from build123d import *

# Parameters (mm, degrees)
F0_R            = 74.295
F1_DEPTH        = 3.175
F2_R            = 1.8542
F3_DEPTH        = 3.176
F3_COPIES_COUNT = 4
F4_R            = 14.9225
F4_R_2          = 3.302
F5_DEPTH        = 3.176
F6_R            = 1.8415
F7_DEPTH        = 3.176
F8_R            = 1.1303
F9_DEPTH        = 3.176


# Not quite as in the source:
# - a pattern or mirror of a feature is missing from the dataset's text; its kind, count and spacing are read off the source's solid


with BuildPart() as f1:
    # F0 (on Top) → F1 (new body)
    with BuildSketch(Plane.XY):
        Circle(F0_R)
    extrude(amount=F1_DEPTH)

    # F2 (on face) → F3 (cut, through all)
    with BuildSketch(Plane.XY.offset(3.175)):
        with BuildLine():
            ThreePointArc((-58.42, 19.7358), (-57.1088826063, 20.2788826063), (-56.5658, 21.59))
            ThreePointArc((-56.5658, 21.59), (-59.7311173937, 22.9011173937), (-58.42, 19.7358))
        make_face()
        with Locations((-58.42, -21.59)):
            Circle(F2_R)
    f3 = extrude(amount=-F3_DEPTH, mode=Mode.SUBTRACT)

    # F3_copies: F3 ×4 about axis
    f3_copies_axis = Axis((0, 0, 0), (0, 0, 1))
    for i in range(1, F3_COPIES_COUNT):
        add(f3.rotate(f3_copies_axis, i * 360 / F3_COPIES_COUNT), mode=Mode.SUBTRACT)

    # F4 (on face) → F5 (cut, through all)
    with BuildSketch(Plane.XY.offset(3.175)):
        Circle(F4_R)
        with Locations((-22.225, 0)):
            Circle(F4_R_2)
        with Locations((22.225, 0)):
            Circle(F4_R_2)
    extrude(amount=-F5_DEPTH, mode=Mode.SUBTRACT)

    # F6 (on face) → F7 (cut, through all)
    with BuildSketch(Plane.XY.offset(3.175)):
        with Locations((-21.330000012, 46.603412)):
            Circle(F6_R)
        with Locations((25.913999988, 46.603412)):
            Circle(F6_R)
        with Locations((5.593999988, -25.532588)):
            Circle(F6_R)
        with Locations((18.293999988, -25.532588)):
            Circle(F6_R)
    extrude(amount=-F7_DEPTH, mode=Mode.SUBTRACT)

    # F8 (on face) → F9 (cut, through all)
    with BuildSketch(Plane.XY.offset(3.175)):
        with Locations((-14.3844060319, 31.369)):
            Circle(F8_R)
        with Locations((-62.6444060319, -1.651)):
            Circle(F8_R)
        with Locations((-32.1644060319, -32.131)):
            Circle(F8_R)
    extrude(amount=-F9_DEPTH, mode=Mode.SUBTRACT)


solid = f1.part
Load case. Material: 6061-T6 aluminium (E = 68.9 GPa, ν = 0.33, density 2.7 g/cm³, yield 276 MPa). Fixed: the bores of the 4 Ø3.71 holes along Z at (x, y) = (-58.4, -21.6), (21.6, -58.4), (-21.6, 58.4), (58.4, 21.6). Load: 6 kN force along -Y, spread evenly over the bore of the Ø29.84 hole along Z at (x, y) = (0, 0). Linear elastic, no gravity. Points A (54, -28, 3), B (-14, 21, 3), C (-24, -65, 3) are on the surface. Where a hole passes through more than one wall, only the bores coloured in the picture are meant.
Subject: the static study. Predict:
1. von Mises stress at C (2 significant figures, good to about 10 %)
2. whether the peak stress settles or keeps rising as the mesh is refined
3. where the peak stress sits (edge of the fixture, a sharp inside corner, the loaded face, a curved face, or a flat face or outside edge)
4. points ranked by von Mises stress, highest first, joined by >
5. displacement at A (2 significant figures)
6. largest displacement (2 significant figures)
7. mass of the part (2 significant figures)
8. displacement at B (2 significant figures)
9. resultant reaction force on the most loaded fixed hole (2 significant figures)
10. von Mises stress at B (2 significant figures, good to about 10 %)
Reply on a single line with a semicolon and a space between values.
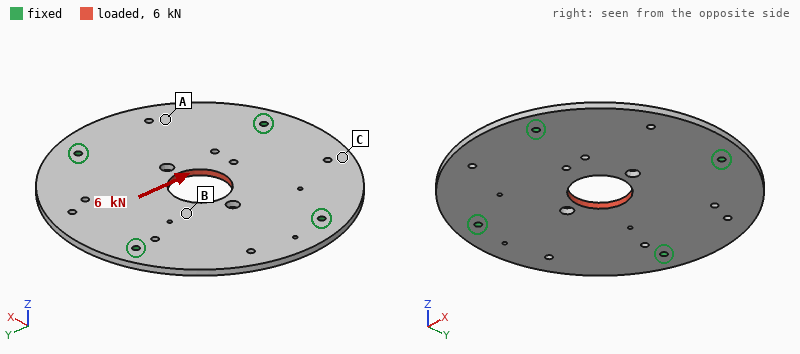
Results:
8.6 MPa; keeps rising; edge of the fixture; B > C > A; 6.2 µm; 19 µm; 140 g; 14 µm; 1.8 kN; 20 MPa
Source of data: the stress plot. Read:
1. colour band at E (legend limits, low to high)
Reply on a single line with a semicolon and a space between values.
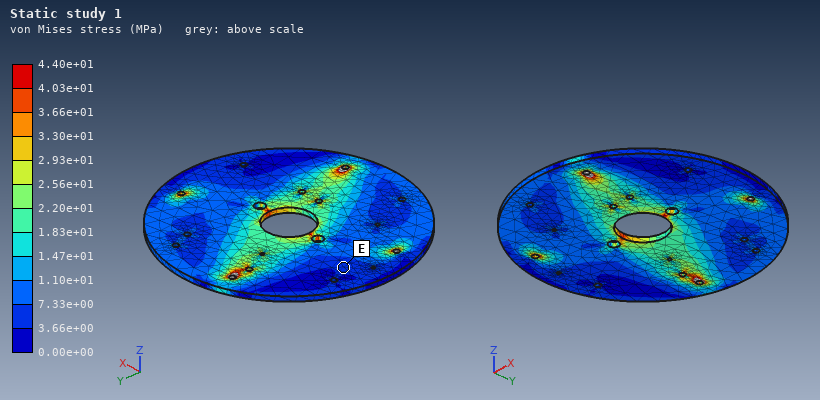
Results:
3.66e+00 to 7.33e+00 MPa
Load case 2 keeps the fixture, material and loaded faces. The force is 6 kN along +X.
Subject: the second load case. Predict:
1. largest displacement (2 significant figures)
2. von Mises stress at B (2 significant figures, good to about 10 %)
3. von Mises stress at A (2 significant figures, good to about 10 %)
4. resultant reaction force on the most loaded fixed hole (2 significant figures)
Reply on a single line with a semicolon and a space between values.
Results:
20 µm; 11 MPa; 6.3 MPa; 1.8 kN
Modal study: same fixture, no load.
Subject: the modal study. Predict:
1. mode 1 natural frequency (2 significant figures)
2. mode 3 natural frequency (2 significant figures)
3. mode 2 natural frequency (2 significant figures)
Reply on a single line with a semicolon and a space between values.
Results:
1500 Hz; 1600 Hz; 1500 Hz
